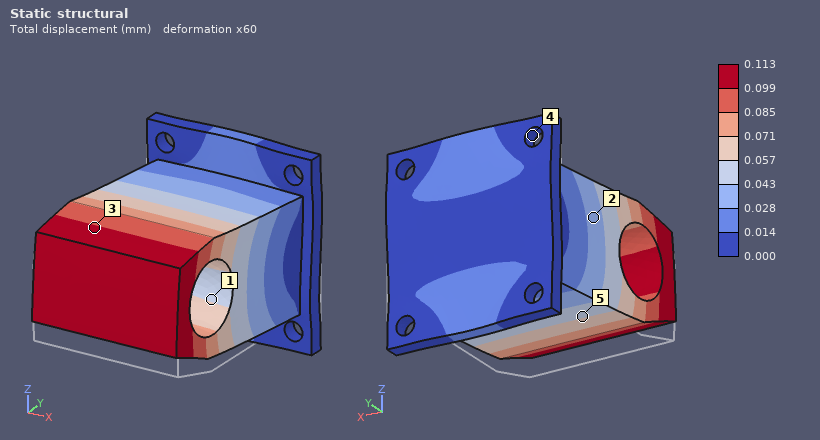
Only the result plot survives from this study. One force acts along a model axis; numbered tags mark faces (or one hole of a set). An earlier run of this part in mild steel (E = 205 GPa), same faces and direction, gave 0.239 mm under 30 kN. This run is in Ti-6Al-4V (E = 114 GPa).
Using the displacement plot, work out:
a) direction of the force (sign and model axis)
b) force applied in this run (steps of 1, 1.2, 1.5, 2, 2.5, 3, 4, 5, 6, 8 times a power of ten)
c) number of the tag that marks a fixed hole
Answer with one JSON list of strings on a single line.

["+Z", "8 kN", "4"]
